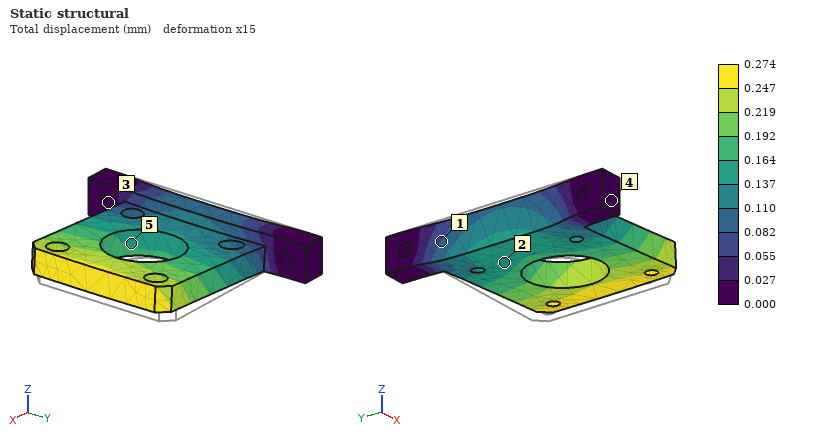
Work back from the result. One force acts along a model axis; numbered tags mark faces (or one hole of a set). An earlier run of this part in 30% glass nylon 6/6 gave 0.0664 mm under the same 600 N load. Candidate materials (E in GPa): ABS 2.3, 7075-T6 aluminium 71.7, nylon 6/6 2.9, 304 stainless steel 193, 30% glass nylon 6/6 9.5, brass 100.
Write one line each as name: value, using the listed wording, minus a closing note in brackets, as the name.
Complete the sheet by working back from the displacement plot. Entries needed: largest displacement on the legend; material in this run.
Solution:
largest displacement on the legend: 0.274 mm
material in this run: ABS
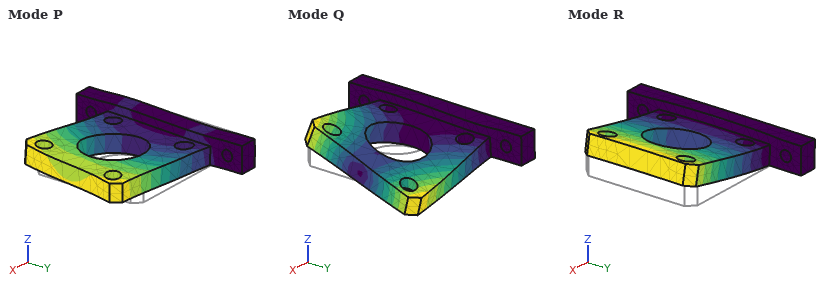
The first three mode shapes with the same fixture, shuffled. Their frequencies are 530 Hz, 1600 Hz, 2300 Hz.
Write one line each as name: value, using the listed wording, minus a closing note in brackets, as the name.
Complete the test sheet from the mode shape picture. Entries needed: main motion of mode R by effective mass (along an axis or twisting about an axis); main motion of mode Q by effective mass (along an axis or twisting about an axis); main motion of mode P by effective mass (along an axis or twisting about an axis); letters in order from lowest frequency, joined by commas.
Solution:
main motion of mode R by effective mass: along Z
main motion of mode Q by effective mass: twisting about X
main motion of mode P by effective mass: along Y
letters in order from lowest frequency, joined by commas: R, Q, P
